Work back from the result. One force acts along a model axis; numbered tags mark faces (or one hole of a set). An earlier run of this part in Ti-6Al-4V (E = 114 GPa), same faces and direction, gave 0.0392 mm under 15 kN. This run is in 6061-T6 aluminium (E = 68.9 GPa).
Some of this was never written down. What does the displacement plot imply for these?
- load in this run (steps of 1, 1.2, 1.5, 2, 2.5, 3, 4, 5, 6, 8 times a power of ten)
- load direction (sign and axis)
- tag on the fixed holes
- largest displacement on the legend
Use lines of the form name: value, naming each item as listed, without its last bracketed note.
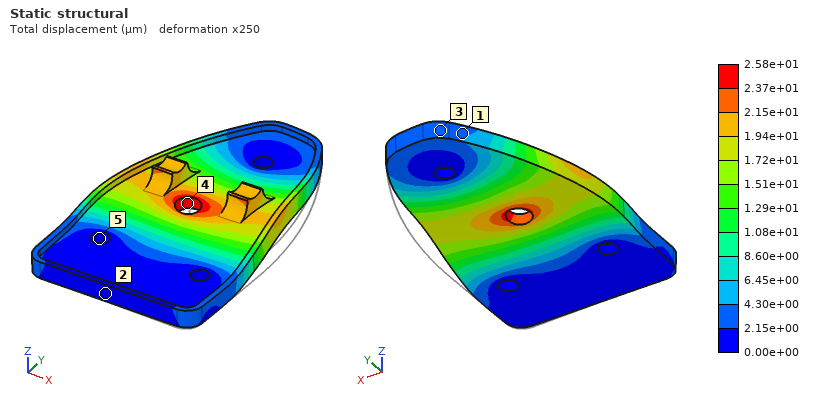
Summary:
load in this run: 6 kN
load direction: -X
tag on the fixed holes: 5
largest displacement on the legend: 2.58e+01 µm
